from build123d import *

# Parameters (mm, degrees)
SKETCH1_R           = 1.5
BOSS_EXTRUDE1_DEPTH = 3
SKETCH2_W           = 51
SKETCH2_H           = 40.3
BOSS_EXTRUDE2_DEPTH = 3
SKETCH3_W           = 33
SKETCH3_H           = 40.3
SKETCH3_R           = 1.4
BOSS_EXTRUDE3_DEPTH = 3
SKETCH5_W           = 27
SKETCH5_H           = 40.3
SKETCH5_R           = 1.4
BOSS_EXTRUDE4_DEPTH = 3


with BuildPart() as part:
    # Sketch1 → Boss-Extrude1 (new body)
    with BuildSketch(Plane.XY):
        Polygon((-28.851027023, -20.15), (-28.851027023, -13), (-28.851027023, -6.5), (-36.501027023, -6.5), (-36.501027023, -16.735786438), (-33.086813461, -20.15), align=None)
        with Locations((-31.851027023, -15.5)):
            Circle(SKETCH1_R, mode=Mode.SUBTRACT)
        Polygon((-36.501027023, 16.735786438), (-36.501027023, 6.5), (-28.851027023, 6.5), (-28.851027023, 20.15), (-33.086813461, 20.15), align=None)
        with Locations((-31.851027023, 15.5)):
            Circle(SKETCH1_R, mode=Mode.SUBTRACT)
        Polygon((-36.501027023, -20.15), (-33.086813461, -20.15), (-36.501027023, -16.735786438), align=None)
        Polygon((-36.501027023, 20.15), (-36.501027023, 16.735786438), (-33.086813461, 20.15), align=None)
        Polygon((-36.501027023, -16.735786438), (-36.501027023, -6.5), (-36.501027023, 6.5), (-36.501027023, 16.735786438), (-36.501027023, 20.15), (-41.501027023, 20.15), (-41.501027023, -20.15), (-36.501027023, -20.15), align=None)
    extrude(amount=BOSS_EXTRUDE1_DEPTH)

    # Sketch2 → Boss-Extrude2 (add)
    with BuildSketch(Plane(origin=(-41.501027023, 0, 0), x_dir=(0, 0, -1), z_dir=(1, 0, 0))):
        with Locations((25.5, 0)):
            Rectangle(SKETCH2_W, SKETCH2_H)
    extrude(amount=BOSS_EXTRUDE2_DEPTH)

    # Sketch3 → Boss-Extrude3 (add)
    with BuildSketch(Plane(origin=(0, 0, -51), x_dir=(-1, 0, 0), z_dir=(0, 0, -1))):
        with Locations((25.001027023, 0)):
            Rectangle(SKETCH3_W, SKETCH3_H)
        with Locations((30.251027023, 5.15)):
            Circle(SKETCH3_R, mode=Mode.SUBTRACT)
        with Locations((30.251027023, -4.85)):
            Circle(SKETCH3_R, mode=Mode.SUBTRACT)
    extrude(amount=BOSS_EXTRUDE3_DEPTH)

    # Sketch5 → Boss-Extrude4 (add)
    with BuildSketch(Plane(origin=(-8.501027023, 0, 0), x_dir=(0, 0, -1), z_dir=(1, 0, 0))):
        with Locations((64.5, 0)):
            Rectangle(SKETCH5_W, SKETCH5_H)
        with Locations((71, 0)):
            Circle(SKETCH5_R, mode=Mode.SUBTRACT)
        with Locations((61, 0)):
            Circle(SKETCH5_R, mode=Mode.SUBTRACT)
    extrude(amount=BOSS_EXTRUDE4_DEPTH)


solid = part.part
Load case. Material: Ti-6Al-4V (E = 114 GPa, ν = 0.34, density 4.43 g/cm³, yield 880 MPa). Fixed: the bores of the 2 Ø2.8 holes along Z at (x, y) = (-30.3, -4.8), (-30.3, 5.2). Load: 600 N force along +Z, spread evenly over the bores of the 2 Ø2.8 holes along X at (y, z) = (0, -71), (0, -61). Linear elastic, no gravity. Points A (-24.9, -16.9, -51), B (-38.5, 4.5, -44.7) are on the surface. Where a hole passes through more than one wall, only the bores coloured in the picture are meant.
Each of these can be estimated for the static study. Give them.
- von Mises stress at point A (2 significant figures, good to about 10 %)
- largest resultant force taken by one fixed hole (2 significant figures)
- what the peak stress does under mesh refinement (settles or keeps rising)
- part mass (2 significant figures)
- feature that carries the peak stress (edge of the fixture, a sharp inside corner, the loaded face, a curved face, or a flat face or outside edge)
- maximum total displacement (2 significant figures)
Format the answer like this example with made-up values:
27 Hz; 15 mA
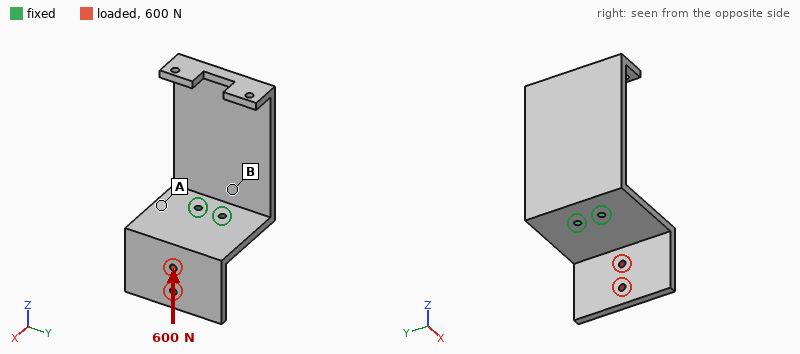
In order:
120 MPa; 300 N; keeps rising; 64 g; edge of the fixture; 0.51 mm
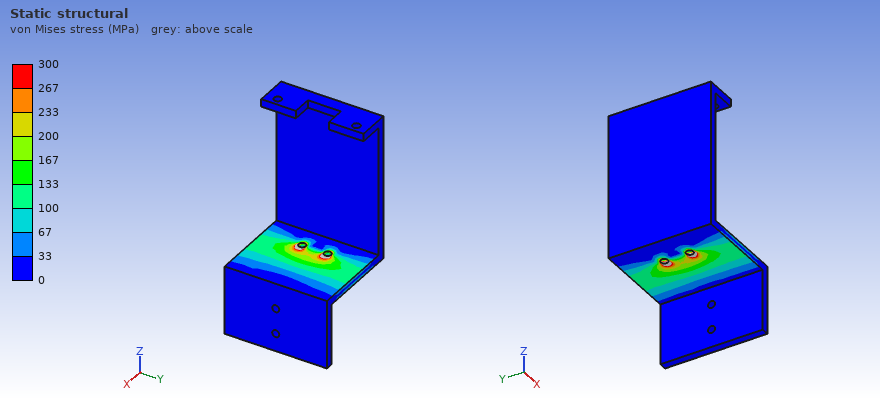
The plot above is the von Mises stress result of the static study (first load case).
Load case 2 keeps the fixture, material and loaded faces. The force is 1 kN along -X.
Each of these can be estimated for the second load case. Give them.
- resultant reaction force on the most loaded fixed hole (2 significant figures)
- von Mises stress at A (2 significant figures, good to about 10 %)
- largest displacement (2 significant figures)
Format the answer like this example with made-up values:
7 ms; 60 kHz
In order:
530 N; 170 MPa; 1.0 mm
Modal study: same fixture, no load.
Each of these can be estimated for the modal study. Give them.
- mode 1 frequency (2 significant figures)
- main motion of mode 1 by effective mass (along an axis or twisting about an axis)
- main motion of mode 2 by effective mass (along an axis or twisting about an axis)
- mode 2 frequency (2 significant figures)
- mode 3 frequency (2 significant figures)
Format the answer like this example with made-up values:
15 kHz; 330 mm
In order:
520 Hz; along X; along Y; 1300 Hz; 1400 Hz
